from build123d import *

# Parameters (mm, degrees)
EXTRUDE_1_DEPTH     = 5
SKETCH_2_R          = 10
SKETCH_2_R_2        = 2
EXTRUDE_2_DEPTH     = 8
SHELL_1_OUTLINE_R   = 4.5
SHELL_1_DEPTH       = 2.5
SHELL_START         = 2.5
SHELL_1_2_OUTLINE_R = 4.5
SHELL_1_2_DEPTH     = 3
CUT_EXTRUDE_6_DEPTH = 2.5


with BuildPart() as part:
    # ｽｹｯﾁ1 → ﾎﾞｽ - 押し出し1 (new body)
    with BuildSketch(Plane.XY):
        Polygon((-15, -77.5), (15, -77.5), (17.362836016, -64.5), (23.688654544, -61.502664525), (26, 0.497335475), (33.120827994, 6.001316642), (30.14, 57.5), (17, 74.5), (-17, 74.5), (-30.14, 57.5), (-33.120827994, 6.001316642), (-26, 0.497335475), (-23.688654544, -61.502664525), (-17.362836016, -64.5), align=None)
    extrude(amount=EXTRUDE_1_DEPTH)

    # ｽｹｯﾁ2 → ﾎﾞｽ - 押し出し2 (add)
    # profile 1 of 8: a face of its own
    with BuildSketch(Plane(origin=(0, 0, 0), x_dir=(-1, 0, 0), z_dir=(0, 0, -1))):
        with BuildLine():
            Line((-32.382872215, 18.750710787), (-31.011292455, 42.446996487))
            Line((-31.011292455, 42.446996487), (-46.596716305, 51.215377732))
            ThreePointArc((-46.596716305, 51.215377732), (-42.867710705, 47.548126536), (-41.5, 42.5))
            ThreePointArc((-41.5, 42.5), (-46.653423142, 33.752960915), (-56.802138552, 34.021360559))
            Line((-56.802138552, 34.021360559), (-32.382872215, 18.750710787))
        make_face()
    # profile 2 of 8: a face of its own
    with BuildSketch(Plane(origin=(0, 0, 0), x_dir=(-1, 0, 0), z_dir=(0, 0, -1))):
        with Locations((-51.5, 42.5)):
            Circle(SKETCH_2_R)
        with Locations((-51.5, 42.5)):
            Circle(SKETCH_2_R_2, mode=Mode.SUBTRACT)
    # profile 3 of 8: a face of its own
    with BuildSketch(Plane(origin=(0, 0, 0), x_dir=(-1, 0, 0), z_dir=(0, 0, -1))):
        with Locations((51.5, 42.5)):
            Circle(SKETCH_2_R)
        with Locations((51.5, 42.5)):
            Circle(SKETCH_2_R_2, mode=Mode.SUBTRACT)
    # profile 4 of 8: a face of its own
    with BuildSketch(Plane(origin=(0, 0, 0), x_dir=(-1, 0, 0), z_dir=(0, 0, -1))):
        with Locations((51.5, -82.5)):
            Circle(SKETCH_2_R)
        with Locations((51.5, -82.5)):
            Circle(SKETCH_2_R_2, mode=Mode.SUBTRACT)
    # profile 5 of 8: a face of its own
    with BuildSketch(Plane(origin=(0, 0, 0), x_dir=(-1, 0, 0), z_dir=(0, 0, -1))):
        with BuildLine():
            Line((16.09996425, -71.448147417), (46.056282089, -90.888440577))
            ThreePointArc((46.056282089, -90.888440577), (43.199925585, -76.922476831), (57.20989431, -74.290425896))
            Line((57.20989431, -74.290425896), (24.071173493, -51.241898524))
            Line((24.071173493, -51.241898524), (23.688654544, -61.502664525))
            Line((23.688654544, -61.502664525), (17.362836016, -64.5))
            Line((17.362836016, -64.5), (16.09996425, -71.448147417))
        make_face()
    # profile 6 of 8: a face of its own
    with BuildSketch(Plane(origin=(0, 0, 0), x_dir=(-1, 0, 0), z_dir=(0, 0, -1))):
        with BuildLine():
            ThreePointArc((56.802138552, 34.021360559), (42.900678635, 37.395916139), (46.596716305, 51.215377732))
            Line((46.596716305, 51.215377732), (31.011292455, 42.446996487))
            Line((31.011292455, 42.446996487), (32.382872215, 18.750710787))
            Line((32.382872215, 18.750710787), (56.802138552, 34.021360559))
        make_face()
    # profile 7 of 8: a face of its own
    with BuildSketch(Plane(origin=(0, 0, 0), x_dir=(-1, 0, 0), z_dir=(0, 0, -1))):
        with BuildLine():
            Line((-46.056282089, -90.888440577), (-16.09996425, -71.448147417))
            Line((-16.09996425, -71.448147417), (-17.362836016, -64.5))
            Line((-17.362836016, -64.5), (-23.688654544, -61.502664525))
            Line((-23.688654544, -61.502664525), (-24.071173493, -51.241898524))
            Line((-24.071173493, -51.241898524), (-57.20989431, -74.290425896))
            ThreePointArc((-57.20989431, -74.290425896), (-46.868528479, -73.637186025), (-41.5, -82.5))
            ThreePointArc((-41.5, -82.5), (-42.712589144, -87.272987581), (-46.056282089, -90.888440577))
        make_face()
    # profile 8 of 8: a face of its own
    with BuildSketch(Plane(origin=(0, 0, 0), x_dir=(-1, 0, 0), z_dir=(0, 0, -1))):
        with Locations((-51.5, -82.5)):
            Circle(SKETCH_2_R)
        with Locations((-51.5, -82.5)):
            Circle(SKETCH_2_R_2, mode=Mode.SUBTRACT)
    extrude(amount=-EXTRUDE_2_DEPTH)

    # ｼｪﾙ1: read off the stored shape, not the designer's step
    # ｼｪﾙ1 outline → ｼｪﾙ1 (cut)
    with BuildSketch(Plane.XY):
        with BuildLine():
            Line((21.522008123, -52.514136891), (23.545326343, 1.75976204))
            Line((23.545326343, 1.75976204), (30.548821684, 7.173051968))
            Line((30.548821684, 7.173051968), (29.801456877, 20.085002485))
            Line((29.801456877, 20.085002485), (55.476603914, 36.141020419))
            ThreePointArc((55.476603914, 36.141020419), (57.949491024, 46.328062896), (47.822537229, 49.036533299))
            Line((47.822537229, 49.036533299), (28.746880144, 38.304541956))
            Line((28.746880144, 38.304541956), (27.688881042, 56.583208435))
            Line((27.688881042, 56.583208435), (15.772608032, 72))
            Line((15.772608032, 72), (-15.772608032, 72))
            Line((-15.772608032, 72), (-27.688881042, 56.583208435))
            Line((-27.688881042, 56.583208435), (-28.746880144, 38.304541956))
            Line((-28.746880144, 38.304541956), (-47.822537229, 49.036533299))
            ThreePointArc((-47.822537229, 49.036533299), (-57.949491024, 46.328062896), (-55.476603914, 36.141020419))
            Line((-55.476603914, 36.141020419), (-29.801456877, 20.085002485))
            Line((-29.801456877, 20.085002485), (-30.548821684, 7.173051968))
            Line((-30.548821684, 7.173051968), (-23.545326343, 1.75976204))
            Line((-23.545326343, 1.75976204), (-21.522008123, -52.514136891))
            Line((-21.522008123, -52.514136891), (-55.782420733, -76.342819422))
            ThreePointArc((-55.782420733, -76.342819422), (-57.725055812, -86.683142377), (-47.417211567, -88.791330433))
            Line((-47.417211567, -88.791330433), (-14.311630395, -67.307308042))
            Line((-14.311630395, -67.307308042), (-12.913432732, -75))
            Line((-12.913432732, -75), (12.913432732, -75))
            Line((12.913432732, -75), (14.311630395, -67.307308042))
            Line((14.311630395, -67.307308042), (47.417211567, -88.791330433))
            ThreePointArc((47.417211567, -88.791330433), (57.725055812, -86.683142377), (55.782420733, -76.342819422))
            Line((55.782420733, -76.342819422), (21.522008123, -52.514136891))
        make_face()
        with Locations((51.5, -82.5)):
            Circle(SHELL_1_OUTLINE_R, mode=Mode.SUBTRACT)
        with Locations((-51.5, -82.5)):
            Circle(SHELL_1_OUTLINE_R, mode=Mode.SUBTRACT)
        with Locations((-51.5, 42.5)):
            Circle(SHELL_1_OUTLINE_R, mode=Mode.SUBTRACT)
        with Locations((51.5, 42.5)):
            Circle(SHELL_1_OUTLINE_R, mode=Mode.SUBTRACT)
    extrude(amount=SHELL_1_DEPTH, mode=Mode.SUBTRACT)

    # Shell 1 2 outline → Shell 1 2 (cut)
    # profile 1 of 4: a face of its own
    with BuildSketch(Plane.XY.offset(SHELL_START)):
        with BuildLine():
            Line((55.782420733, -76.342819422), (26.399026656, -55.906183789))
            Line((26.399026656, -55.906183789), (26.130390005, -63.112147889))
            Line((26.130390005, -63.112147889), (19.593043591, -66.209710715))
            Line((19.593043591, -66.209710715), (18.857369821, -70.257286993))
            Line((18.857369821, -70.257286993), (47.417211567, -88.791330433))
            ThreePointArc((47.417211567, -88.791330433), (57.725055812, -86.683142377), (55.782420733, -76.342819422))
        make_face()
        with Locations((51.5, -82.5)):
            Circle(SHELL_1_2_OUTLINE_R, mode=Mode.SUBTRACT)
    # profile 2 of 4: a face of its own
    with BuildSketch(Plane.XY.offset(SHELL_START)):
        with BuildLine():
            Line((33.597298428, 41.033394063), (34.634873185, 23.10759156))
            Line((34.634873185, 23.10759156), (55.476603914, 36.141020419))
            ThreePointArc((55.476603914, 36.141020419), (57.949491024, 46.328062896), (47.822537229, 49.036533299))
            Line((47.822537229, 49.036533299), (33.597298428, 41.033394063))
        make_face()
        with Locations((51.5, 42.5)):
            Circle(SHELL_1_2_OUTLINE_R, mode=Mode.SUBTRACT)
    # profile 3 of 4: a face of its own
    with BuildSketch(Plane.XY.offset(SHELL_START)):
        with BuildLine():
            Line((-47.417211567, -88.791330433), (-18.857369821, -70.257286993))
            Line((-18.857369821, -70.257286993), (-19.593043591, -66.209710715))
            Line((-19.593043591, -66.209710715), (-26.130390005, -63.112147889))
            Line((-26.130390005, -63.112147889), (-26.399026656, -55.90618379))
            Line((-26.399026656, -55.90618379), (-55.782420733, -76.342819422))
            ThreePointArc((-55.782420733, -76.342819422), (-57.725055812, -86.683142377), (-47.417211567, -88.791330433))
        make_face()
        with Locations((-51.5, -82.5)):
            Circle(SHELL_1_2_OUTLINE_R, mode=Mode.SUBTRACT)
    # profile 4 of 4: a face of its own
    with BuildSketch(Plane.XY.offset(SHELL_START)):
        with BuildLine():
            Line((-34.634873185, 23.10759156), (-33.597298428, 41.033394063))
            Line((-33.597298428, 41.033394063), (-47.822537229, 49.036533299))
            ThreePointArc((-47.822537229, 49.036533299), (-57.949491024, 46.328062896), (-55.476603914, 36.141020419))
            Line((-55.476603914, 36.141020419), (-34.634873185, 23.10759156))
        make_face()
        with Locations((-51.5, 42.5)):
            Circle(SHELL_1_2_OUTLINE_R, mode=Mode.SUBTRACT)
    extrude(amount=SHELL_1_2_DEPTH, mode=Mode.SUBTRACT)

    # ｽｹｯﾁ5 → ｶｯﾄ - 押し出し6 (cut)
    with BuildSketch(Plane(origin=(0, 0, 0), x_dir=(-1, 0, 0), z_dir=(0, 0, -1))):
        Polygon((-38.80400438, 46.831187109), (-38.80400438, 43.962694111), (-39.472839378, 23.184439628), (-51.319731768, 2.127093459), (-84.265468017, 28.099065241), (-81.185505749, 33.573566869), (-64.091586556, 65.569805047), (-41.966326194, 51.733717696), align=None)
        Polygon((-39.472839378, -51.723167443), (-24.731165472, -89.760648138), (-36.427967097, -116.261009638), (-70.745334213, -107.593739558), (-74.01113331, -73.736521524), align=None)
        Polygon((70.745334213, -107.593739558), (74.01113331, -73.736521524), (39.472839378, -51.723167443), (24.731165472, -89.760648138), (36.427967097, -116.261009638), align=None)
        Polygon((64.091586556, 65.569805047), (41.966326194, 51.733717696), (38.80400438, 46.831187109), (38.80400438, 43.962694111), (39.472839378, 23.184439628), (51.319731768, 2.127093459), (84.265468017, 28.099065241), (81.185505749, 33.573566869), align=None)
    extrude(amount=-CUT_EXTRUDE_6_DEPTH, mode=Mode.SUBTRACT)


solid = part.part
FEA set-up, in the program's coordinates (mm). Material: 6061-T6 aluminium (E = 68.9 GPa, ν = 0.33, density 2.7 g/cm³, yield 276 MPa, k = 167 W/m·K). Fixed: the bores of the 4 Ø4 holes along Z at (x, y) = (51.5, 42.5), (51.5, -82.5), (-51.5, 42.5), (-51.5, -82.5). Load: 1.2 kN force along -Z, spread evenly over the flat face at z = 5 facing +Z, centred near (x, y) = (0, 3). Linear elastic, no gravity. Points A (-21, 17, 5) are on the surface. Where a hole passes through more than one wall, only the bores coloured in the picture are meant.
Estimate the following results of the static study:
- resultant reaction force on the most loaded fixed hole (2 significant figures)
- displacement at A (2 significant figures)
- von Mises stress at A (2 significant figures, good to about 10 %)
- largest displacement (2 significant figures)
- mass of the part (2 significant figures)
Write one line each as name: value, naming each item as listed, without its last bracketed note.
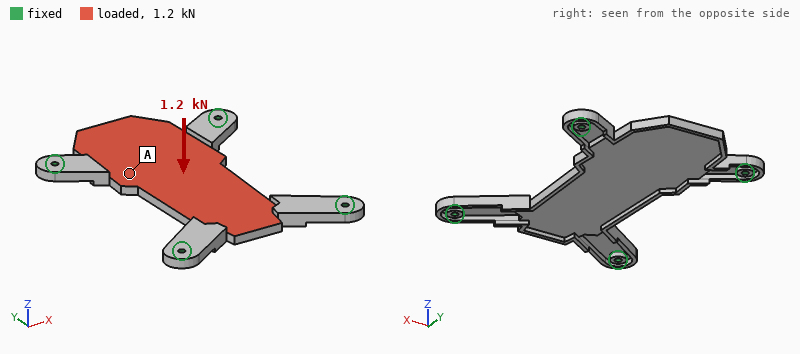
resultant reaction force on the most loaded fixed hole: 1.8 kN
displacement at A: 0.32 mm
von Mises stress at A: 17 MPa
largest displacement: 0.54 mm
mass of the part: 92 g
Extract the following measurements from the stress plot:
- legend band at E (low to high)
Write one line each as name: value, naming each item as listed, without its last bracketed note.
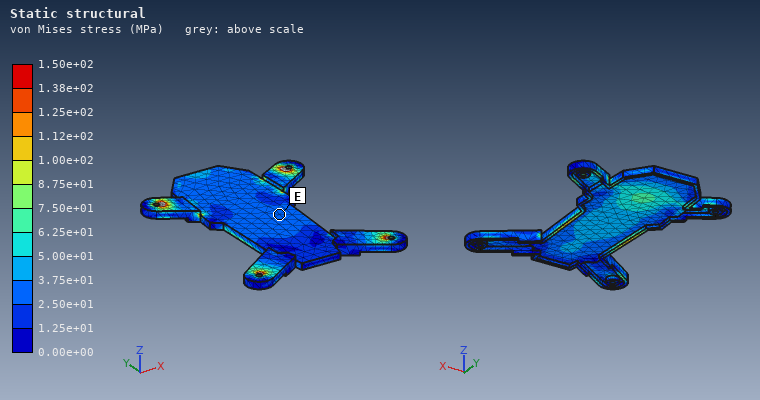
legend band at E: 2.50e+01 to 3.75e+01 MPa
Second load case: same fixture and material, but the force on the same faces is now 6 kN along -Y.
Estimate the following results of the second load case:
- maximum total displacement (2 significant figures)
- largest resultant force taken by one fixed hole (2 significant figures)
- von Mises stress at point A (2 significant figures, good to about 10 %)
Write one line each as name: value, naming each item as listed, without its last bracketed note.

maximum total displacement: 0.19 mm
largest resultant force taken by one fixed hole: 2.1 kN
von Mises stress at point A: 48 MPa
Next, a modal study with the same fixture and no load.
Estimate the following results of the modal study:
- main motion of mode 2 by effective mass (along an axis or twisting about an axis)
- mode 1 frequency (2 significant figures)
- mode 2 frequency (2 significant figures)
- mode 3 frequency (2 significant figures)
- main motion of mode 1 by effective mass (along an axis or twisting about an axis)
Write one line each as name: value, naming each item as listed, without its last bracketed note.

main motion of mode 2 by effective mass: along Z
mode 1 frequency: 1100 Hz
mode 2 frequency: 1200 Hz
mode 3 frequency: 1800 Hz
main motion of mode 1 by effective mass: along Z
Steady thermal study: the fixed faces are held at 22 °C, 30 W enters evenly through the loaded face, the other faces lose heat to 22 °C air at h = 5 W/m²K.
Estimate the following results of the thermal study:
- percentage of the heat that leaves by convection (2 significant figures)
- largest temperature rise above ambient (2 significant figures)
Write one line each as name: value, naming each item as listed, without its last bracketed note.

percentage of the heat that leaves by convection: 5.8 %
largest temperature rise above ambient: 29 K
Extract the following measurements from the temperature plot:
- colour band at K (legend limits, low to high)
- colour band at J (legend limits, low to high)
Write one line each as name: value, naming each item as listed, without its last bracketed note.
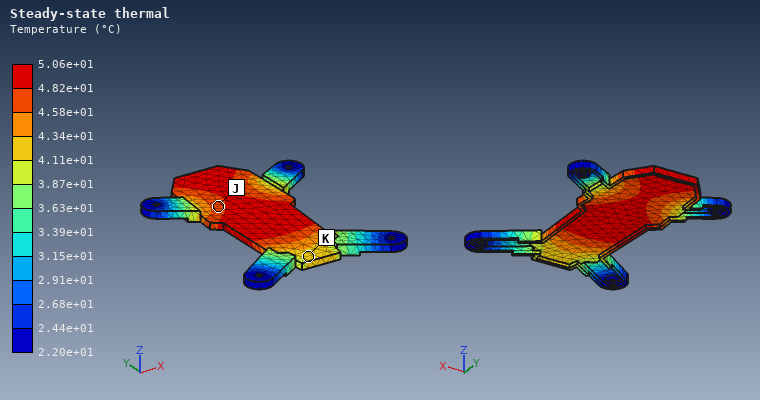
colour band at K: 4.11e+01 to 4.34e+01 °C
colour band at J: 4.58e+01 to 4.82e+01 °C
